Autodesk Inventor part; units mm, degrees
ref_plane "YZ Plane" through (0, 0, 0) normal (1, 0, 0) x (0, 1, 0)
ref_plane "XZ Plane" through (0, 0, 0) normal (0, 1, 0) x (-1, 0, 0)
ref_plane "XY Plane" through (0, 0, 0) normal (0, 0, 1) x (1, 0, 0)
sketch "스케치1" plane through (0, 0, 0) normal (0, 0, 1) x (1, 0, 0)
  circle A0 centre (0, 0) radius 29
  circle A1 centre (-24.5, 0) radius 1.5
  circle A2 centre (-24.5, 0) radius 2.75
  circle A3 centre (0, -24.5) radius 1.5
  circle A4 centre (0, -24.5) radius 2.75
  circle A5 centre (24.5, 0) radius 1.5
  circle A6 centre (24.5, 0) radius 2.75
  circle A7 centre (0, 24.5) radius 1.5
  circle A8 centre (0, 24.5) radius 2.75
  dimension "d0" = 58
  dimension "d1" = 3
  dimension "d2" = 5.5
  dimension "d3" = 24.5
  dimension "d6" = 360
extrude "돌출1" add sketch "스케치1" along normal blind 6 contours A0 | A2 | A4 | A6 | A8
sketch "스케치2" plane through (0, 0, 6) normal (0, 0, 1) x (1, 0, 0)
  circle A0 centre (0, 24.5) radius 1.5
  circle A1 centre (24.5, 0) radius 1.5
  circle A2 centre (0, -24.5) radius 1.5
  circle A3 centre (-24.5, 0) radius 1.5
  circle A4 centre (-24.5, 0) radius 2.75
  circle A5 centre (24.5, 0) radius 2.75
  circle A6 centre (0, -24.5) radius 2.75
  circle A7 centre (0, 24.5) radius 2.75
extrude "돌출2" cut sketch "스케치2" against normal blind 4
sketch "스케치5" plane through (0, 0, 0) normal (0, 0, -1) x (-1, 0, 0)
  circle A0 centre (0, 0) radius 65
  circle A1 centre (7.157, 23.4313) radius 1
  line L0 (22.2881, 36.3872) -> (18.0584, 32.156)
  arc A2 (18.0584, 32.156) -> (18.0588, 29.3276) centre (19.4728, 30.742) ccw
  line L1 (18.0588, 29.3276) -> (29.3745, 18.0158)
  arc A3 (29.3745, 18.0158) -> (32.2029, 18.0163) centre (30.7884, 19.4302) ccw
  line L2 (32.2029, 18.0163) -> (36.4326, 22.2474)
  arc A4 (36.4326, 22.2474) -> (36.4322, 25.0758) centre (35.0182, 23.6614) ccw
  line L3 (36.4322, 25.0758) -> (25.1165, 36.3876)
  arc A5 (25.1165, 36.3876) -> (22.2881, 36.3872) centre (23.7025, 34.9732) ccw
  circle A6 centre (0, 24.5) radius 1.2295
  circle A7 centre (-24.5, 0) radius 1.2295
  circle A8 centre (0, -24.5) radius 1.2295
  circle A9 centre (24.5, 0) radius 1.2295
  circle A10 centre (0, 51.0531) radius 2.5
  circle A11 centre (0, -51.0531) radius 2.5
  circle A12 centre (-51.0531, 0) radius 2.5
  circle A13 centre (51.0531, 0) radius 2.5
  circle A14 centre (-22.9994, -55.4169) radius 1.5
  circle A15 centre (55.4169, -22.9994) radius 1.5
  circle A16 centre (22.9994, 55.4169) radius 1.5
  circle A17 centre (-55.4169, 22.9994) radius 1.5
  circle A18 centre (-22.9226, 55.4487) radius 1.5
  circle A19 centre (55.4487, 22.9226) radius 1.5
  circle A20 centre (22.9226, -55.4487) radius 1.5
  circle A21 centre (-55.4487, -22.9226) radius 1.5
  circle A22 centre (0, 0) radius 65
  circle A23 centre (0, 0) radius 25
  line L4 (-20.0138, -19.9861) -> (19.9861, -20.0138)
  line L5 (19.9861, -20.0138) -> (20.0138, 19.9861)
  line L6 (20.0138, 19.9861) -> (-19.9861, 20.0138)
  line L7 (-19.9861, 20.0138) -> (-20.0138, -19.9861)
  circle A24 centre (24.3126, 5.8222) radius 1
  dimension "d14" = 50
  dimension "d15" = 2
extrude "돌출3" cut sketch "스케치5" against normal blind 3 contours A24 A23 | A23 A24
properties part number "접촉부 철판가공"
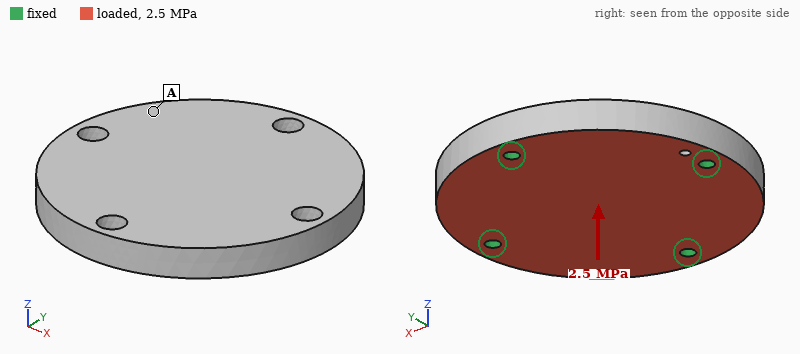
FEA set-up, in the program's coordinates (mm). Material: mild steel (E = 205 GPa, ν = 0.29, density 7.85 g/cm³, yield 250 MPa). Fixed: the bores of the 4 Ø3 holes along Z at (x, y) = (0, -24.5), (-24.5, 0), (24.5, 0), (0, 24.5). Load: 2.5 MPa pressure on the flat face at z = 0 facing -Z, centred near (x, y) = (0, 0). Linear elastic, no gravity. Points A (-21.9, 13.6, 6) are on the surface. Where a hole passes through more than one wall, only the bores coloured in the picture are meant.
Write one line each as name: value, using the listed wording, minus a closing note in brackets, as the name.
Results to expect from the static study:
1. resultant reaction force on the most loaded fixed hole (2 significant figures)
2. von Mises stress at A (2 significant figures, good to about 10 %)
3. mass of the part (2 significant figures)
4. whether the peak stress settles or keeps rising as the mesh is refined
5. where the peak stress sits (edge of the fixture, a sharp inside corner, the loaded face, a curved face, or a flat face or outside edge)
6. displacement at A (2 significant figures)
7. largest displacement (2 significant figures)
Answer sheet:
resultant reaction force on the most loaded fixed hole: 1.9 kN
von Mises stress at A: 33 MPa
mass of the part: 120 g
whether the peak stress settles or keeps rising as the mesh is refined: keeps rising
where the peak stress sits: edge of the fixture
displacement at A: 6.7 µm
largest displacement: 13 µm
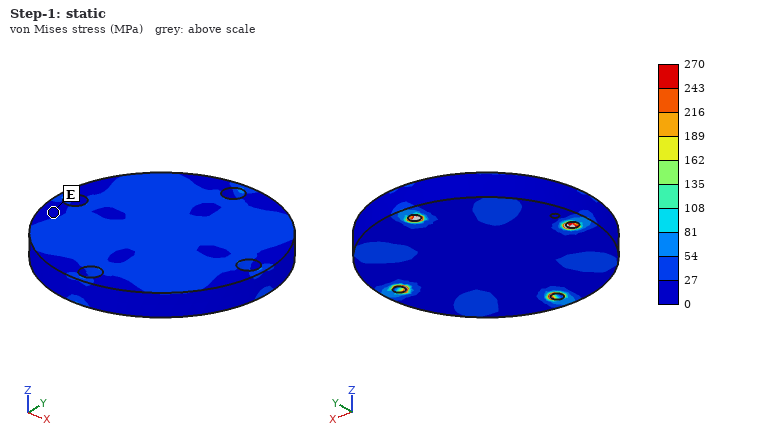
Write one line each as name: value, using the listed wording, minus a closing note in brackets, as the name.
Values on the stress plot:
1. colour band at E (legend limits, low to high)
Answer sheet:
colour band at E: 0 to 27 MPa
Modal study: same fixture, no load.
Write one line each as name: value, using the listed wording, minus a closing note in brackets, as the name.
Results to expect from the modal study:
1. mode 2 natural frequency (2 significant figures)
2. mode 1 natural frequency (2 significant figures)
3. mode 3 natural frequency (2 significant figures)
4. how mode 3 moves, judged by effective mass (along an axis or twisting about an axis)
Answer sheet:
mode 2 natural frequency: 13 kHz
mode 1 natural frequency: 12 kHz
mode 3 natural frequency: 14 kHz
how mode 3 moves, judged by effective mass: twisting about Y
